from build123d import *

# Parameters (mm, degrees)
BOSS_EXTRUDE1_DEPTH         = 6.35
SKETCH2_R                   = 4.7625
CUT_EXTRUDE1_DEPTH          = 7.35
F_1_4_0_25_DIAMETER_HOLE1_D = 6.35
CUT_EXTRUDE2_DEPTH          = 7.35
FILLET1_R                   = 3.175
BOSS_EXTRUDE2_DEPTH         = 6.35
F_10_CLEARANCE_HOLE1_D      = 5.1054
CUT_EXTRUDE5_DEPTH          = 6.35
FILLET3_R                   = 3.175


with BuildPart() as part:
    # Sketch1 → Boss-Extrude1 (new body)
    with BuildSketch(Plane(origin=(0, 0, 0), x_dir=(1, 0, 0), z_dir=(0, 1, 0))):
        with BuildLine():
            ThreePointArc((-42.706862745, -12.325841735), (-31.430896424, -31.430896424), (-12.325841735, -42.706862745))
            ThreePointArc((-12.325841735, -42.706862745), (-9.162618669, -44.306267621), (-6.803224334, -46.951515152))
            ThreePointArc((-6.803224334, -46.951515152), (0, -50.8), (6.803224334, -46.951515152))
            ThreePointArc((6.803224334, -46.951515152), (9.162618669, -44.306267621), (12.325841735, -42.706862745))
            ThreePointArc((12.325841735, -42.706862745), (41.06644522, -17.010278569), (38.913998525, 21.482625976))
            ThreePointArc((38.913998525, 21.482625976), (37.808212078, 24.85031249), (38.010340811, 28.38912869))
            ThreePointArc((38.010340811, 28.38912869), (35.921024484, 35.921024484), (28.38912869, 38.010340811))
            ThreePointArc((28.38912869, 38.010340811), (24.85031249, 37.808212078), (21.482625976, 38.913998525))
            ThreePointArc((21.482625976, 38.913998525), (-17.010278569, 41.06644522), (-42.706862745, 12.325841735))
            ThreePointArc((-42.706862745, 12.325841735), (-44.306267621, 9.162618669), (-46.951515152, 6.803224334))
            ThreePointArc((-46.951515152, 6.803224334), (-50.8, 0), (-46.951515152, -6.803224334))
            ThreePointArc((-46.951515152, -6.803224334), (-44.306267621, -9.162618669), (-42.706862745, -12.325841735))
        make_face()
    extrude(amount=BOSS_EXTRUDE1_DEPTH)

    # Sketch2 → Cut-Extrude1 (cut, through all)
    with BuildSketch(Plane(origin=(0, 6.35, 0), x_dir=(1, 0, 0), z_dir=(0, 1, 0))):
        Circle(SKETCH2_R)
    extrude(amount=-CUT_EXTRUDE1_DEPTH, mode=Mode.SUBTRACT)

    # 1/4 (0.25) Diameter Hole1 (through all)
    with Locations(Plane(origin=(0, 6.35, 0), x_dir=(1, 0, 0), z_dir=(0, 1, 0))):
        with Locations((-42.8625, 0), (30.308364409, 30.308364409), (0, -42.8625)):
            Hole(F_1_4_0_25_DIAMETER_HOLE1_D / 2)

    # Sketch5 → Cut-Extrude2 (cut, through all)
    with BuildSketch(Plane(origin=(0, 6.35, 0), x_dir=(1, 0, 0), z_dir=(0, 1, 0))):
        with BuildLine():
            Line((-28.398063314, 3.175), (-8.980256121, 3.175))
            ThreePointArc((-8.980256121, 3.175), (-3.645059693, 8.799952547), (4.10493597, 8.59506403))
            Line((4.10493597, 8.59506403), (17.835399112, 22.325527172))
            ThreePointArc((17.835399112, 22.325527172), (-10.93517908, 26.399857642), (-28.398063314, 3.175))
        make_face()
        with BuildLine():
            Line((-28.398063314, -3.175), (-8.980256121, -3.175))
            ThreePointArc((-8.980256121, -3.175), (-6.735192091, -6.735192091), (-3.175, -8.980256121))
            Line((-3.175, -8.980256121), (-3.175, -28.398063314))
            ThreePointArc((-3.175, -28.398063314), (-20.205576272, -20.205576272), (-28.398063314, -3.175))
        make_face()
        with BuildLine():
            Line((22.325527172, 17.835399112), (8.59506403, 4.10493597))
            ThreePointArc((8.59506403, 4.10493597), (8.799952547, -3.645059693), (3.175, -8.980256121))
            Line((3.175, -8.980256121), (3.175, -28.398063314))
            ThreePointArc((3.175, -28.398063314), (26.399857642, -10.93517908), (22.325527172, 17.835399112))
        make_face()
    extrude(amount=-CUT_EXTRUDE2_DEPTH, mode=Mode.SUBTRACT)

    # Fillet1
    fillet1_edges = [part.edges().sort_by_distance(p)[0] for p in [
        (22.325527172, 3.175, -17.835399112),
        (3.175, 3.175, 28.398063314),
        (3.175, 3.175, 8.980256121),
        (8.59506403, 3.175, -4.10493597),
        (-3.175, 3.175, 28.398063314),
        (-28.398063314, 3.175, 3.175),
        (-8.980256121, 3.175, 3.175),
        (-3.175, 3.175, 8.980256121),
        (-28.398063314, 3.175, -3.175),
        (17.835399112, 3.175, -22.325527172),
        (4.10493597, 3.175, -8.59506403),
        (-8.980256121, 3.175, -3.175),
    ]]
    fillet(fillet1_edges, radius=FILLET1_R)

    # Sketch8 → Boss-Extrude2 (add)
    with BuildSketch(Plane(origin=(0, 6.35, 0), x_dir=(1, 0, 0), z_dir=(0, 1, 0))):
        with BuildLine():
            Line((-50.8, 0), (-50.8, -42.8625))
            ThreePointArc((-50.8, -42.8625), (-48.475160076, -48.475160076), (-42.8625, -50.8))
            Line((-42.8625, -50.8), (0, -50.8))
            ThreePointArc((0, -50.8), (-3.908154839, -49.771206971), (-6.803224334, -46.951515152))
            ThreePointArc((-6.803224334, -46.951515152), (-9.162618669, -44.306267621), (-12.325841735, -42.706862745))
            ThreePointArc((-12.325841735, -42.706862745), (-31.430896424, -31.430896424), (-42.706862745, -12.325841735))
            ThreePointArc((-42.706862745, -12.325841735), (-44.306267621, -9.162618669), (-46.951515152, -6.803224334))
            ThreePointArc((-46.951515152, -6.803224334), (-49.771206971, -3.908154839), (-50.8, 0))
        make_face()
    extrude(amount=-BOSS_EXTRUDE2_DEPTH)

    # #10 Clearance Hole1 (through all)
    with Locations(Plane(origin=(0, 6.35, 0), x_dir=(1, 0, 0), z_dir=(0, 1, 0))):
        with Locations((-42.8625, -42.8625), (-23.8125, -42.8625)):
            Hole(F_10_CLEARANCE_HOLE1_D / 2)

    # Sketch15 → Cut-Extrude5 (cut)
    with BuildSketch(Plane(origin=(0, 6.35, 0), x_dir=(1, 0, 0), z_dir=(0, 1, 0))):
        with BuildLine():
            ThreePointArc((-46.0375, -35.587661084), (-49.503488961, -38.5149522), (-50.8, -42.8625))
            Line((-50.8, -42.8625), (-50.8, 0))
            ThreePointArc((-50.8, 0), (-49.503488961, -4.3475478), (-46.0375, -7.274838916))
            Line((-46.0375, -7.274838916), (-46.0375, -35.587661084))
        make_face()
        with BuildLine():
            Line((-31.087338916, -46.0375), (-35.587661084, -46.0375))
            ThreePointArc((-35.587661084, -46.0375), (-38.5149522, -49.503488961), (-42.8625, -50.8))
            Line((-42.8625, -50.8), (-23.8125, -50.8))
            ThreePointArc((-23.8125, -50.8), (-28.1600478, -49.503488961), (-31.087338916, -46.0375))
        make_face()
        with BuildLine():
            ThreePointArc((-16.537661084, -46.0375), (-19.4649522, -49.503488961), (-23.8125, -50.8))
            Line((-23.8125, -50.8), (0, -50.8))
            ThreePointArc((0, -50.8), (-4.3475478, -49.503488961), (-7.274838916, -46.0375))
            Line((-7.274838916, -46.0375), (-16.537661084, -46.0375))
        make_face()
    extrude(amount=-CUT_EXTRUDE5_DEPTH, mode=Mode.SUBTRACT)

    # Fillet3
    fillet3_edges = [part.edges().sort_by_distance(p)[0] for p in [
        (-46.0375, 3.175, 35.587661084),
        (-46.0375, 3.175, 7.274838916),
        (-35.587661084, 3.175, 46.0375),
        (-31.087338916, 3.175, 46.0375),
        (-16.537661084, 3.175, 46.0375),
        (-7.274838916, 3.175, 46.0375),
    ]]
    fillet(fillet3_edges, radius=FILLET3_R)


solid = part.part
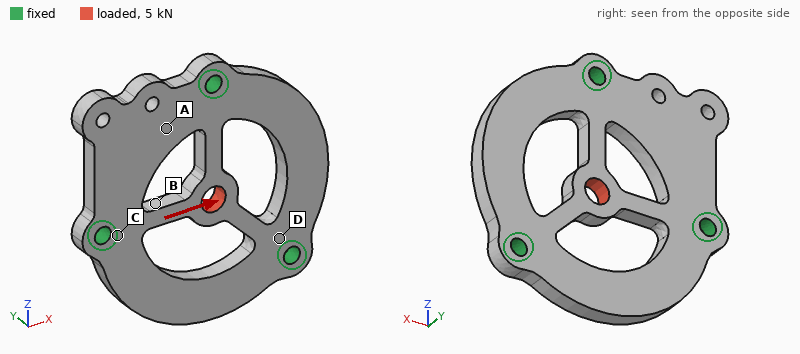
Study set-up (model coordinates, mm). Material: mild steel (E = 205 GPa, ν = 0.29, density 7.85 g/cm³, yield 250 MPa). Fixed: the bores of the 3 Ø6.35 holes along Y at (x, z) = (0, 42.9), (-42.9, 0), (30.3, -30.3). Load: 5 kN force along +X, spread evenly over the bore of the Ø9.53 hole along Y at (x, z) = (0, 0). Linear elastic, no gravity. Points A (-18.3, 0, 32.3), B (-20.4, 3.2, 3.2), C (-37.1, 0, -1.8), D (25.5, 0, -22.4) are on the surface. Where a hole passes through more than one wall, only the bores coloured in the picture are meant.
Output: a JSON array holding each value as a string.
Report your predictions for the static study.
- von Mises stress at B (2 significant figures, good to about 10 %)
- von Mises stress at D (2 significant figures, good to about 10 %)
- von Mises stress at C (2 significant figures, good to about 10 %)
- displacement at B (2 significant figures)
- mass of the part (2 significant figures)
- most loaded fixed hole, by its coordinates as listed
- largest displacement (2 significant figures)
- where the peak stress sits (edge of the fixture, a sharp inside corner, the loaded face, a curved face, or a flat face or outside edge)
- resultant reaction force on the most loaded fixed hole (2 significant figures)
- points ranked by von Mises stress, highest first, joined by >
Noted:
["78 MPa", "30 MPa", "49 MPa", "5.3 µm", "250 g", "(-42.9, 0)", "23 µm", "a curved face", "3.2 kN", "B > C > D > A"]
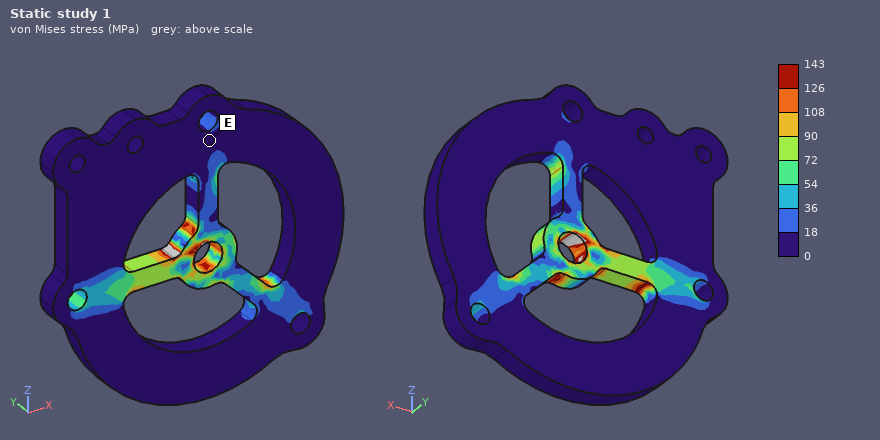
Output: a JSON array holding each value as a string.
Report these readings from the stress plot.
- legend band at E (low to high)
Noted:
["0 to 18 MPa"]
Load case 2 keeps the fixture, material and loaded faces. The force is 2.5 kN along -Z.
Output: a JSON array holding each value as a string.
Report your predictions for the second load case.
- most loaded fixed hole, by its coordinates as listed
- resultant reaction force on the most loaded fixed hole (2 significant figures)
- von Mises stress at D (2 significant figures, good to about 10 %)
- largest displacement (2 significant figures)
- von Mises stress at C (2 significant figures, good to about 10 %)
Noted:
["(0, 42.9)", "1.6 kN", "7.8 MPa", "11 µm", "7.2 MPa"]
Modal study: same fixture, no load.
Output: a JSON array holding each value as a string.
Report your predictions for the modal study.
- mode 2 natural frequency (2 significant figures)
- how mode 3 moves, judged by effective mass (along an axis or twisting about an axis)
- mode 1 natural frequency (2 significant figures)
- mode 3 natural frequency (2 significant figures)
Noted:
["3800 Hz", "along Y", "3700 Hz", "4000 Hz"]
